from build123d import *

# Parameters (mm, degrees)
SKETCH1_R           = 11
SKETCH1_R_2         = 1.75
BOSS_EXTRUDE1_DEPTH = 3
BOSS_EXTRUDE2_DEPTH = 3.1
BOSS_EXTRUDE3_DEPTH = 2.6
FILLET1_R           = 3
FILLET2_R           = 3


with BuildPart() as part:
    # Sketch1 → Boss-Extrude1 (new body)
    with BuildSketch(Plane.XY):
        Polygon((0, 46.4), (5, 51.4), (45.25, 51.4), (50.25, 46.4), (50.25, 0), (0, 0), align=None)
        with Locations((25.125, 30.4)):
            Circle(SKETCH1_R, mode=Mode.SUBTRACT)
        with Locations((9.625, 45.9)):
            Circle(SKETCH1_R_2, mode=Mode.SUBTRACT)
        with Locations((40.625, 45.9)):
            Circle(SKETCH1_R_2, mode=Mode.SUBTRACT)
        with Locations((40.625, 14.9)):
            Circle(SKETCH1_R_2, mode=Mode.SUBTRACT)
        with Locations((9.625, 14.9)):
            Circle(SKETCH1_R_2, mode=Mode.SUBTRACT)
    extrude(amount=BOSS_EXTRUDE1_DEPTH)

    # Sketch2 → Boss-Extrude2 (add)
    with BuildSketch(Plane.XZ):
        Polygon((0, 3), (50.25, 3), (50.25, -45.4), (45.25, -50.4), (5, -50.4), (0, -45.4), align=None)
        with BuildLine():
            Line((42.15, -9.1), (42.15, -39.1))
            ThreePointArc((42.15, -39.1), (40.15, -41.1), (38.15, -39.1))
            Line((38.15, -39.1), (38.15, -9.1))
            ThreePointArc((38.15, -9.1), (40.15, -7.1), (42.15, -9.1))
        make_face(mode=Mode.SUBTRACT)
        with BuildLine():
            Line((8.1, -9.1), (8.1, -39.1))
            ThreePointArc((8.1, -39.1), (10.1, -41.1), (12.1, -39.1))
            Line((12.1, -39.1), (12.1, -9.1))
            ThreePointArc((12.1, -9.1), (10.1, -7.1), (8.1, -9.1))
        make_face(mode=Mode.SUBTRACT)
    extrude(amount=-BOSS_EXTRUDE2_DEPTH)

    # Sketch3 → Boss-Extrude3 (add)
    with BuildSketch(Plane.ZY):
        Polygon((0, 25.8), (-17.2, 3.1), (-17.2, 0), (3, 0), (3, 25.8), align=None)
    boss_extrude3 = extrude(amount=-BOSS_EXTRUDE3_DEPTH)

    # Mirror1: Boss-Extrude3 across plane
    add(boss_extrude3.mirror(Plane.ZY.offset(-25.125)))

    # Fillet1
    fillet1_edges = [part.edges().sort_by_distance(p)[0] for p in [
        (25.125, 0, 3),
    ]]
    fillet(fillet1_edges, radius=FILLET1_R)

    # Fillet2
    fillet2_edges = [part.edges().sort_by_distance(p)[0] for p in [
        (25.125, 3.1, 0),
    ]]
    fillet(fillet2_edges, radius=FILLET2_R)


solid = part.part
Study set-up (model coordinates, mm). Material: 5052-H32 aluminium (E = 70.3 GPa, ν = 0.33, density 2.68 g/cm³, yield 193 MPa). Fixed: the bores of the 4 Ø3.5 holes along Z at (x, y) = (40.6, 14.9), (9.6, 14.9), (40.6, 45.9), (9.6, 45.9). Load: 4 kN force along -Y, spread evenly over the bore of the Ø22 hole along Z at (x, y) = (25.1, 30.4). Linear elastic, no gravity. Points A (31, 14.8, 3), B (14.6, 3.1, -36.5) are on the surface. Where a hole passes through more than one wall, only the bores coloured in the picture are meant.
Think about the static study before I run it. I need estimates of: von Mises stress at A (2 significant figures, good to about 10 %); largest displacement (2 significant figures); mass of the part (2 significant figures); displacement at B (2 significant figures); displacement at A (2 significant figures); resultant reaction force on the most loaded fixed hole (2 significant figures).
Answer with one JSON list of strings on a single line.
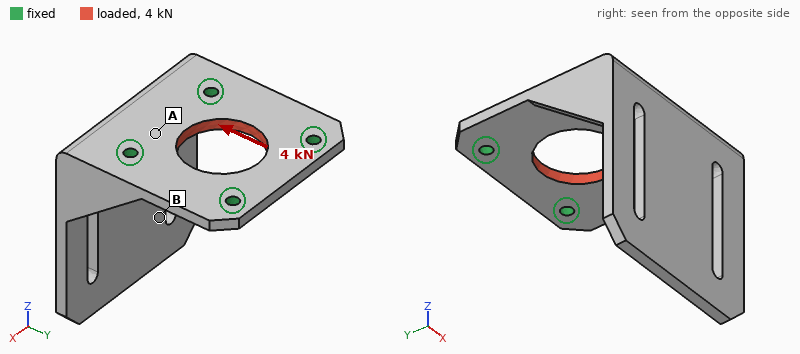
["15 MPa", "12 µm", "39 g", "4.5 µm", "4.6 µm", "1.0 kN"]
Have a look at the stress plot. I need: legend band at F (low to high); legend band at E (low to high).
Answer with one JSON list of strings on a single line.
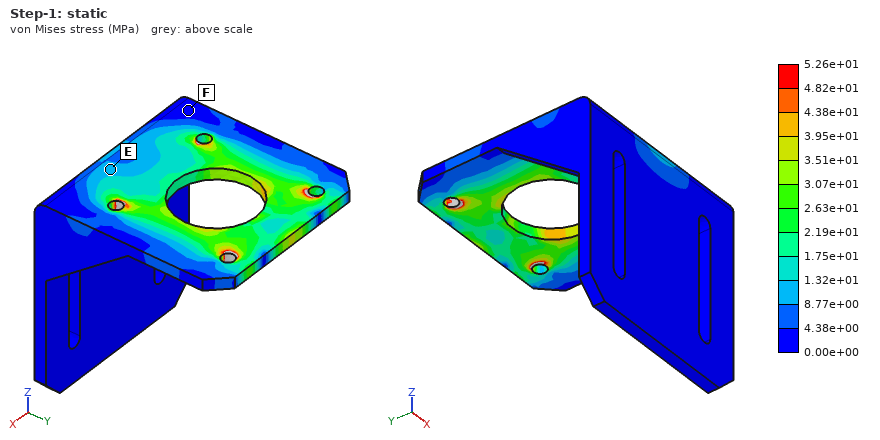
["0.00e+00 to 4.38e+00 MPa", "8.77e+00 to 1.32e+01 MPa"]
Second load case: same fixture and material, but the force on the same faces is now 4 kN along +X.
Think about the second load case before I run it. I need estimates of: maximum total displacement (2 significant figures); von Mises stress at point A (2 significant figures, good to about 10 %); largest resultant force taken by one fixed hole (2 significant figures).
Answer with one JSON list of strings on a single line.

["9.0 µm", "20 MPa", "1.0 kN"]
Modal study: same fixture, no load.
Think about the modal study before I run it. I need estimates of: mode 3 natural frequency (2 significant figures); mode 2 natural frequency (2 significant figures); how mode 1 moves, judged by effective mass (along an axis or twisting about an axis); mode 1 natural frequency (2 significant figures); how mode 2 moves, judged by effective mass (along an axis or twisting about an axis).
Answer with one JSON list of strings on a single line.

["3600 Hz", "2200 Hz", "along Y", "1100 Hz", "along X"]
